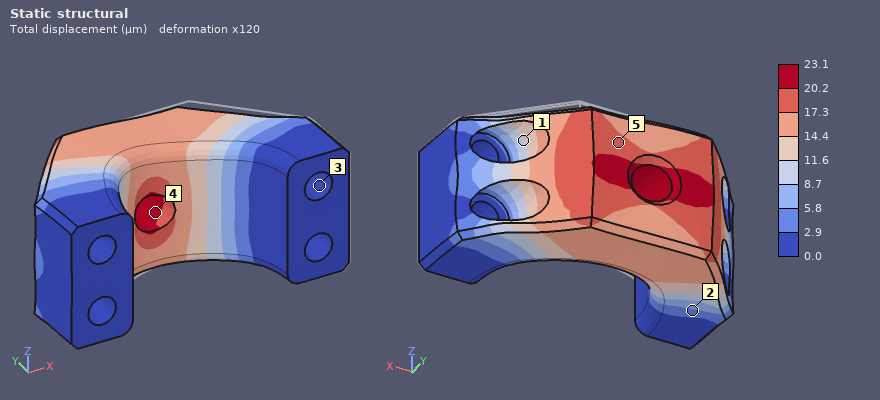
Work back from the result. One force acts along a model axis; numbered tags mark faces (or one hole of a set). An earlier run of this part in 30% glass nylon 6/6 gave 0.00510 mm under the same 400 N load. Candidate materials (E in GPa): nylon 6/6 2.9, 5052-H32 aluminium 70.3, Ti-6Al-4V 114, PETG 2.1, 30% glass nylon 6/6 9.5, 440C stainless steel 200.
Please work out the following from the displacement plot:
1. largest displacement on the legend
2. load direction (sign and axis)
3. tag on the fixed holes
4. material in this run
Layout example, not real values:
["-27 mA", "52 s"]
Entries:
["23.1 µm", "-X", "3", "PETG"]
